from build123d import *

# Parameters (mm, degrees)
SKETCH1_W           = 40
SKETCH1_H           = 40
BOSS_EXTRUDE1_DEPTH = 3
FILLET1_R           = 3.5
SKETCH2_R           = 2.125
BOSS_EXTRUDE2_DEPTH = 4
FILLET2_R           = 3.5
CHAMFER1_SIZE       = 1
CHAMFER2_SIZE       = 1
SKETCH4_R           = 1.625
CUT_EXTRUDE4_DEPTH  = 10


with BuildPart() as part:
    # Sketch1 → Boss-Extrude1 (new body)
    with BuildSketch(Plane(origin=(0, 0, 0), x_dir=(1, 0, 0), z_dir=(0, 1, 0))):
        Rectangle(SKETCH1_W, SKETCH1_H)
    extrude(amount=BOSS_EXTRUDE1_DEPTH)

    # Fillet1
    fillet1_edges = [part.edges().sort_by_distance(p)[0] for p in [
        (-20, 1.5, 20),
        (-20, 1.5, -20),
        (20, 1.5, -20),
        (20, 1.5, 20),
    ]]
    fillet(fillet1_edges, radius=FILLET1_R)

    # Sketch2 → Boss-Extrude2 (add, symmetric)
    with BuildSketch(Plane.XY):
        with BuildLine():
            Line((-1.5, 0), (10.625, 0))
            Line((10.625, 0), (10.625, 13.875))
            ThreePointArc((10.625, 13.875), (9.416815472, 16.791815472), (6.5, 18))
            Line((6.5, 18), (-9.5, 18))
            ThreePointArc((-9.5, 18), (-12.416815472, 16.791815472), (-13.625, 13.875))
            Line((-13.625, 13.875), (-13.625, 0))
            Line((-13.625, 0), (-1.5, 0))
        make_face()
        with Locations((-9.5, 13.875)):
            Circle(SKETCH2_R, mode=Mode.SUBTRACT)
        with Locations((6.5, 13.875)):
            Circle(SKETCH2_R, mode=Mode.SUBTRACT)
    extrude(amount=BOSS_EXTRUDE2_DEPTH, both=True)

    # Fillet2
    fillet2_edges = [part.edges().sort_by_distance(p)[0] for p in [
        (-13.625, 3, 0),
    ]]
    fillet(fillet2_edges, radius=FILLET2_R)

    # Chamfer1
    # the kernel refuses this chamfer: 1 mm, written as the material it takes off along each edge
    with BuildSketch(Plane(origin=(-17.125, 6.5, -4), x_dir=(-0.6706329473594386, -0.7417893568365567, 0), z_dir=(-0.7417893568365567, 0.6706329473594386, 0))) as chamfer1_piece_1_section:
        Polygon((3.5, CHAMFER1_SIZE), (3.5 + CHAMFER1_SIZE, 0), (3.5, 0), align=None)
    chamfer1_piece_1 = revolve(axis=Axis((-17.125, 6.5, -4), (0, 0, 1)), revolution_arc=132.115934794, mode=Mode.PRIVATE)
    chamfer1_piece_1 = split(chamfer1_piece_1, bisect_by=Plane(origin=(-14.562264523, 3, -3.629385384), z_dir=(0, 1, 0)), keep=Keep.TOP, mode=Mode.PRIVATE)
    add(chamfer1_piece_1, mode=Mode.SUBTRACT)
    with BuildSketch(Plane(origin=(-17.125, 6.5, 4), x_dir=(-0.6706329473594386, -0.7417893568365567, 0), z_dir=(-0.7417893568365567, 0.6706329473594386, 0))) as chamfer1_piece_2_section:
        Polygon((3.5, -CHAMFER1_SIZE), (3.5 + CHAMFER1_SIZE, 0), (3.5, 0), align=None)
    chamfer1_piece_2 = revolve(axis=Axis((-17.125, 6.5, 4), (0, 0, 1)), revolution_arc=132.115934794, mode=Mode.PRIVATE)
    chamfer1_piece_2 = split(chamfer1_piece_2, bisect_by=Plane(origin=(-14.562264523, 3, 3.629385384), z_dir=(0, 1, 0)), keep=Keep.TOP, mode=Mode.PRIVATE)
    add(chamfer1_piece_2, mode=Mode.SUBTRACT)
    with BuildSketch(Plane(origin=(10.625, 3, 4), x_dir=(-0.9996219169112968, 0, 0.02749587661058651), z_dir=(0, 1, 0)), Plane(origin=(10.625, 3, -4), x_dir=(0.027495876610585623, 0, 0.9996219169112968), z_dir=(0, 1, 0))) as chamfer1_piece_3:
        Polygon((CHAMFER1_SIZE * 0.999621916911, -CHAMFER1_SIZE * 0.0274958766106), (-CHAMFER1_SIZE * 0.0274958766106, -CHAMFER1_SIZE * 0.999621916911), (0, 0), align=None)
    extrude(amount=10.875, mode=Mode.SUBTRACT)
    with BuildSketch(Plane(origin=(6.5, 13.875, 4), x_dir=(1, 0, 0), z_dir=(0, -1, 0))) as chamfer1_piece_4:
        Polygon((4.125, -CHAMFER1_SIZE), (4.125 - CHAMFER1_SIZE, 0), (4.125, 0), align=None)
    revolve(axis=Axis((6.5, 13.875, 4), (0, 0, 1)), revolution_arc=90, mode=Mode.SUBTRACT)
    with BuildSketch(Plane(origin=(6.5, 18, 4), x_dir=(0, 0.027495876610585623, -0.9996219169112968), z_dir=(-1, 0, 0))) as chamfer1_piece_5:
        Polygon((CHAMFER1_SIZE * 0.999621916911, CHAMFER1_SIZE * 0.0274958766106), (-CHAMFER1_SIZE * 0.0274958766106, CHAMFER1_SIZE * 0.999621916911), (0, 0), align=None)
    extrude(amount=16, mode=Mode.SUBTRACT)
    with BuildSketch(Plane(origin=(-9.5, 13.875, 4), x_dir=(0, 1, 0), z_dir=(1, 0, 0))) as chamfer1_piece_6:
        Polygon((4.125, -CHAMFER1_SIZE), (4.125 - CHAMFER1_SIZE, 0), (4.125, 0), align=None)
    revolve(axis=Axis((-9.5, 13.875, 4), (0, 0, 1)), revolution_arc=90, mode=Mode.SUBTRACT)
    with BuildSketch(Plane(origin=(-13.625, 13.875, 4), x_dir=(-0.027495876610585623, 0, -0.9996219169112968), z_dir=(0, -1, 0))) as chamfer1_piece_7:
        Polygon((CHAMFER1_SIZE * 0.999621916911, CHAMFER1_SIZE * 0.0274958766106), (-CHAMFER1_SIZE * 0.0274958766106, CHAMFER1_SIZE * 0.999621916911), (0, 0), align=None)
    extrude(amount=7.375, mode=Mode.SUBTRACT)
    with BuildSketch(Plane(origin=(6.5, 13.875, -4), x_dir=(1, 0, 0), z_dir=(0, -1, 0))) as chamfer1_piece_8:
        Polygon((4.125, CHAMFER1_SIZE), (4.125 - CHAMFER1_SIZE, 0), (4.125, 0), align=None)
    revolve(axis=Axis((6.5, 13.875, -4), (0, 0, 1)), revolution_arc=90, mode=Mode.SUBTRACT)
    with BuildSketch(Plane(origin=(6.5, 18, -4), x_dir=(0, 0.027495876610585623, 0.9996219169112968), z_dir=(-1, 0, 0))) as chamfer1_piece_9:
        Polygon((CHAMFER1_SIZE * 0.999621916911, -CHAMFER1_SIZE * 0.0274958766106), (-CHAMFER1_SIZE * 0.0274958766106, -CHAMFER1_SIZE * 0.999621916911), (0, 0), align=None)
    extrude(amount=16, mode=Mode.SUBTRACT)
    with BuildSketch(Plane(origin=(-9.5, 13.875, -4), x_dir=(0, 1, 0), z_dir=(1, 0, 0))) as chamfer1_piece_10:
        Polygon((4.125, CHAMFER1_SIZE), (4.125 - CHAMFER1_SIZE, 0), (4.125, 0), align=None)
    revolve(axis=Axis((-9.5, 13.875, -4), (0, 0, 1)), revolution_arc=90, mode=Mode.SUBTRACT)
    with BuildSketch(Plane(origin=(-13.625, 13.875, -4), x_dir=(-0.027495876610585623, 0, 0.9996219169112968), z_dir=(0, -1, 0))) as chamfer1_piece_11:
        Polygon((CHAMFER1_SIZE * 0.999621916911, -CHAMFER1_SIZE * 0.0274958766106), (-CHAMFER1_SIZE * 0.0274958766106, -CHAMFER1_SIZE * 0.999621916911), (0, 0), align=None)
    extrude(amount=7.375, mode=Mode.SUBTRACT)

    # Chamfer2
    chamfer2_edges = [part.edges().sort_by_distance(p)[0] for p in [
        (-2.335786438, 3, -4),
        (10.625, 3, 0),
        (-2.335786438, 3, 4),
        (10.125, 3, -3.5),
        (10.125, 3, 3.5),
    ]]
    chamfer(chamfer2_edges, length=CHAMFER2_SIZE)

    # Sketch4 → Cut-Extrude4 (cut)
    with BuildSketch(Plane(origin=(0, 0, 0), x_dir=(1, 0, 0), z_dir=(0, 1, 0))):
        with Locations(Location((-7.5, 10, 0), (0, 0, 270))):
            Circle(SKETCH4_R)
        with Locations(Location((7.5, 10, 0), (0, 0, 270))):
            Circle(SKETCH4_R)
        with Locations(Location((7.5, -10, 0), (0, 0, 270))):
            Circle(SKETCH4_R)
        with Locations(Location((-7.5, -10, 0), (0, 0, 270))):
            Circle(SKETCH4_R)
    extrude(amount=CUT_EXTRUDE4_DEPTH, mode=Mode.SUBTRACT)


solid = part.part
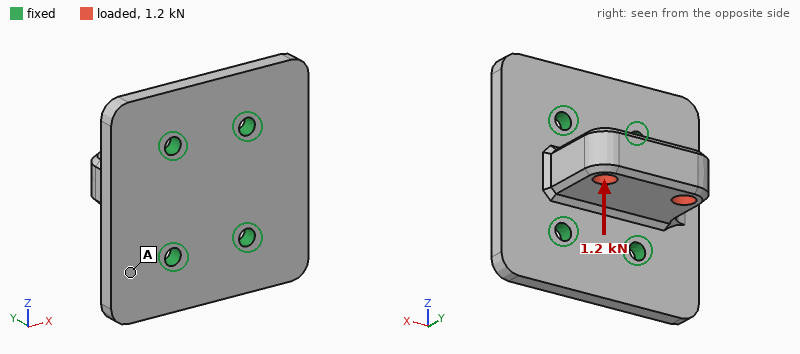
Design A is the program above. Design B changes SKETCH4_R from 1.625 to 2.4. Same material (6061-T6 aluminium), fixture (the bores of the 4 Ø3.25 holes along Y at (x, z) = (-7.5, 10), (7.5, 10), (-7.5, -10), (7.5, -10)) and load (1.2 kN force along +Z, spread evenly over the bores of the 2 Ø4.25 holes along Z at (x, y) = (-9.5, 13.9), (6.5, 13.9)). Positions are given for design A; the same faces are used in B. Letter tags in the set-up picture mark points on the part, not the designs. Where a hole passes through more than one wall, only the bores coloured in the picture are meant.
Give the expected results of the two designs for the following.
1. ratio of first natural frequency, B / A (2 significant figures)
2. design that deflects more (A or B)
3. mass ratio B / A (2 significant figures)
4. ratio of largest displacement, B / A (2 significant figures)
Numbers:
1.2
A
0.98
0.88
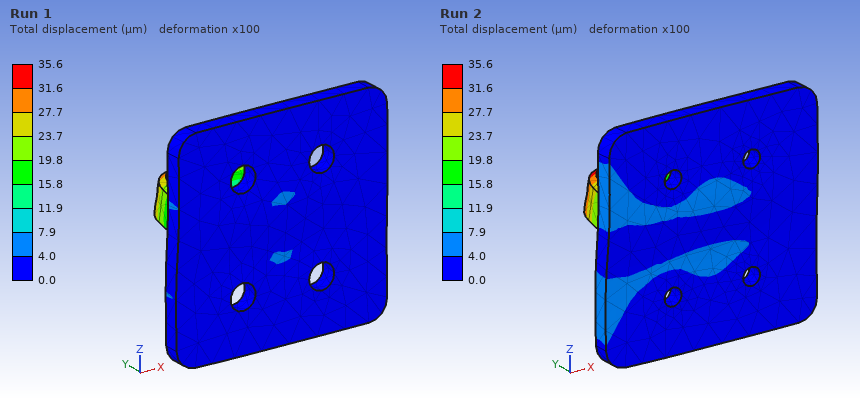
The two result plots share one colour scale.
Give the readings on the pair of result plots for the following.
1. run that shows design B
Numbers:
Run 1
